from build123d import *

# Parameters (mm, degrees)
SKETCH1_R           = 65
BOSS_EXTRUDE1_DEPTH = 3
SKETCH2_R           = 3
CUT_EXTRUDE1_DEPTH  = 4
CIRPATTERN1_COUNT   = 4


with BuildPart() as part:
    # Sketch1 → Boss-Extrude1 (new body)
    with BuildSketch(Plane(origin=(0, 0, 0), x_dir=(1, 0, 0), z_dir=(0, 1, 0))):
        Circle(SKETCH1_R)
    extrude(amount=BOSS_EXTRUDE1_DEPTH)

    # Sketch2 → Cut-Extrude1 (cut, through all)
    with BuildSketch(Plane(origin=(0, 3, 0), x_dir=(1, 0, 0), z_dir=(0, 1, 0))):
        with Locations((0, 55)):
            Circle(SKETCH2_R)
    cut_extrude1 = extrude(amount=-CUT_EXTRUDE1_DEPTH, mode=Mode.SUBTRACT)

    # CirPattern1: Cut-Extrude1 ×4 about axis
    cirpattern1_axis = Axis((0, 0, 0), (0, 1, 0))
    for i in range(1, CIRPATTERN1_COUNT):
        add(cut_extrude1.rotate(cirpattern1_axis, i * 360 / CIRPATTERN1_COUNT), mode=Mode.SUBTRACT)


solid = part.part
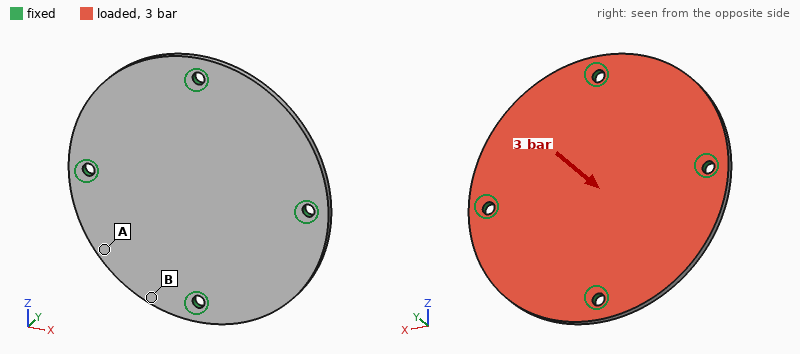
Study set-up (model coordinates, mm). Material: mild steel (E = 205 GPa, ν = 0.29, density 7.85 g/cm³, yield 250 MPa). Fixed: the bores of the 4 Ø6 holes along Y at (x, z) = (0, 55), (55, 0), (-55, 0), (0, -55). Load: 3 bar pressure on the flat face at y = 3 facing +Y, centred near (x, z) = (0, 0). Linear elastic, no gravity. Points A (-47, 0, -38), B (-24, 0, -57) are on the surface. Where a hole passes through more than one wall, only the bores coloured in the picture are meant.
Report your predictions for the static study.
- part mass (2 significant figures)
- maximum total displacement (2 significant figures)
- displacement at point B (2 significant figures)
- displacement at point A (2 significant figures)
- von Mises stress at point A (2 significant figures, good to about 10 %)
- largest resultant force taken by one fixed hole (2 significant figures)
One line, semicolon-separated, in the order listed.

310 g; 0.13 mm; 0.040 mm; 0.078 mm; 48 MPa; 990 N
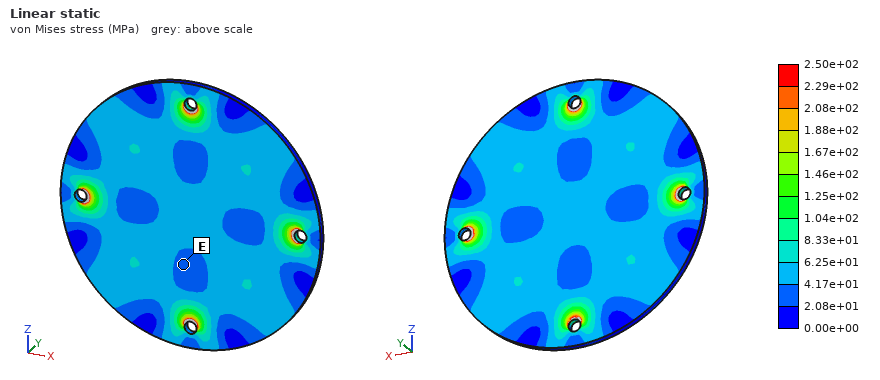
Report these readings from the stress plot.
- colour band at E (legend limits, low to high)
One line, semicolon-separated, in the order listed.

2.08e+01 to 4.17e+01 MPa
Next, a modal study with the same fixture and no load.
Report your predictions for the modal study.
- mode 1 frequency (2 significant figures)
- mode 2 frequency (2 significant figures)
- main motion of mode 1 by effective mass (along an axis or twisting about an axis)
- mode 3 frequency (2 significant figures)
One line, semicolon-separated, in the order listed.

1900 Hz; 2100 Hz; along Y; 2200 Hz
